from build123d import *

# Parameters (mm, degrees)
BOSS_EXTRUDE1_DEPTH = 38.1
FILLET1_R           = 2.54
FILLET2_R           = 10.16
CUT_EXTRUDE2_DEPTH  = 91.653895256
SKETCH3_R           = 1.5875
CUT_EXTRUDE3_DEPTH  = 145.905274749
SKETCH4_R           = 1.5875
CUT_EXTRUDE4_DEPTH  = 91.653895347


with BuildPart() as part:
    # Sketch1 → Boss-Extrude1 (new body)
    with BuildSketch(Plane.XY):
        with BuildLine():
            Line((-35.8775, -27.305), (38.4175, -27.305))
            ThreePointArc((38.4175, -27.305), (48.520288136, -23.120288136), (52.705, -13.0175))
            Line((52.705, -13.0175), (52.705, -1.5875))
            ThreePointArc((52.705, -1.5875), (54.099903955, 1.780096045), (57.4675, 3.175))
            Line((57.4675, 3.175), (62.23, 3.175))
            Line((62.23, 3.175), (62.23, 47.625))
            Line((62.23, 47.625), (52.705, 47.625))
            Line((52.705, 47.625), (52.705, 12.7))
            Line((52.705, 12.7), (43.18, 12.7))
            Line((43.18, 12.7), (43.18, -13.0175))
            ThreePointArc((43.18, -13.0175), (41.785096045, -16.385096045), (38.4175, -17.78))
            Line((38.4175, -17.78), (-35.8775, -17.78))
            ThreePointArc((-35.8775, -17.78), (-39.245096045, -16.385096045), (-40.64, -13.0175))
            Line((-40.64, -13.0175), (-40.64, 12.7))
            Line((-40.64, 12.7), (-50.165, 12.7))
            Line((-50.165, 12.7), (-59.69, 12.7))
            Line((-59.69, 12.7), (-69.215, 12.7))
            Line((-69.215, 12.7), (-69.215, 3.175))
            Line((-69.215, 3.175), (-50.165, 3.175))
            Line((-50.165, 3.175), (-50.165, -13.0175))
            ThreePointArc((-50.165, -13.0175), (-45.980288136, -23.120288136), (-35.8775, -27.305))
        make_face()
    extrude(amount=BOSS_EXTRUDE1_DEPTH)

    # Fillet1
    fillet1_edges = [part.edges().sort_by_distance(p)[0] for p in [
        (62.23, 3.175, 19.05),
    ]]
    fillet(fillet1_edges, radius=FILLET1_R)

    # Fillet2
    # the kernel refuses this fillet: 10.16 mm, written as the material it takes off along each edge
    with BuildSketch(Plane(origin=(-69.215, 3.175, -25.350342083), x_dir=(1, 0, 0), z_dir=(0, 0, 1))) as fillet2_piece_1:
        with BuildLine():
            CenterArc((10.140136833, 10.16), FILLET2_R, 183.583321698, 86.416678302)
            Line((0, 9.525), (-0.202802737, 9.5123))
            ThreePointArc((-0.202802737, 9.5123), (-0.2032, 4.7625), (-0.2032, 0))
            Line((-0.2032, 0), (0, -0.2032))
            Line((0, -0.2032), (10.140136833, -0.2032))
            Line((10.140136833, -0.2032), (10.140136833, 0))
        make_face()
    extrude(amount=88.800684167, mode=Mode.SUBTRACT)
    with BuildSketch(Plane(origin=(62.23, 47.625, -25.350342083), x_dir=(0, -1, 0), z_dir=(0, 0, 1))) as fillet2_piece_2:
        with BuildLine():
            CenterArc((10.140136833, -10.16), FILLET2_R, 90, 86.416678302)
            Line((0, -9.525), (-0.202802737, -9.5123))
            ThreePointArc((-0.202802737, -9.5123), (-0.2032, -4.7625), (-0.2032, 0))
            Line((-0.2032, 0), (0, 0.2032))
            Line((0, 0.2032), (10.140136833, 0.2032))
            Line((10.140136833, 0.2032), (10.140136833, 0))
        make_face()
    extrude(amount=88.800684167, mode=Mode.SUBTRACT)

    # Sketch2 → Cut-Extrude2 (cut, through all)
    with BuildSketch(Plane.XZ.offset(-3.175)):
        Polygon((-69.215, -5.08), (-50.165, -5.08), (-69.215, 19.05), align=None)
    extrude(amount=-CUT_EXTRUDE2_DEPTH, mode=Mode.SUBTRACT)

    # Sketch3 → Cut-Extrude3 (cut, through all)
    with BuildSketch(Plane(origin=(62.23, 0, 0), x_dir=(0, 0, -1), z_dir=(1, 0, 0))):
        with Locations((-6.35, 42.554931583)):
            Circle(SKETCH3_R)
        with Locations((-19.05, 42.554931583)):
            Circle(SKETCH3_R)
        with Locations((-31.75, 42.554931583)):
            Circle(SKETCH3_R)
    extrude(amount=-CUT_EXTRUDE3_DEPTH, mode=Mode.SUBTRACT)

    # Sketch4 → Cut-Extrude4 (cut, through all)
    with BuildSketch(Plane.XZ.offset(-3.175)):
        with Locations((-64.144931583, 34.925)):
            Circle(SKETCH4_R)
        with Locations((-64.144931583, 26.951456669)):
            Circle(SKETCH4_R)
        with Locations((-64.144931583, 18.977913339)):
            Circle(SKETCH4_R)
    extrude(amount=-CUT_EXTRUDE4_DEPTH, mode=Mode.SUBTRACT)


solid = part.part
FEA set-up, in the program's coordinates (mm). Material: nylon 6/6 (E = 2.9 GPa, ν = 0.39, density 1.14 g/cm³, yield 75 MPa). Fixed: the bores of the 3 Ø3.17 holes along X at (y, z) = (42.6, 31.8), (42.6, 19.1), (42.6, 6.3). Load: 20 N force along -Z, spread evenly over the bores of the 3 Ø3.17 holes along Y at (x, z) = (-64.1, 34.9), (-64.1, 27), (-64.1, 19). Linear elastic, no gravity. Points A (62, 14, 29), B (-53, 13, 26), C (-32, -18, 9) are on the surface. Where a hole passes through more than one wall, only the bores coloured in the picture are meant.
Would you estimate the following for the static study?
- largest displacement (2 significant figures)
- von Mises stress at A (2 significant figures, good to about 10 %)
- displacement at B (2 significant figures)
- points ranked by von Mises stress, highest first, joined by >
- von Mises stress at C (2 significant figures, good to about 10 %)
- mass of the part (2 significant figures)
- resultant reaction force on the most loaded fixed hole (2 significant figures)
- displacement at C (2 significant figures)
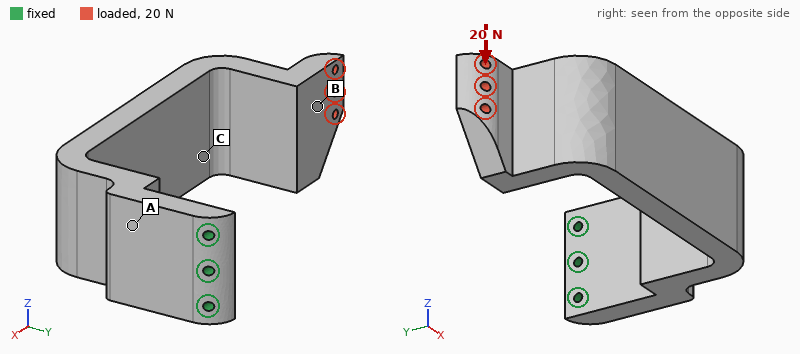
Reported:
1.7 mm
2.9 MPa
1.5 mm
A > C > B
0.98 MPa
87 g
78 N
1.0 mm
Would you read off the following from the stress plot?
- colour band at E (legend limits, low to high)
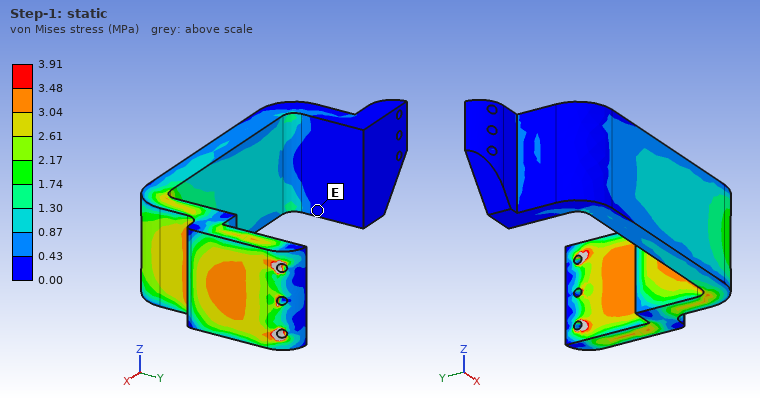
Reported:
0.00 to 0.43 MPa
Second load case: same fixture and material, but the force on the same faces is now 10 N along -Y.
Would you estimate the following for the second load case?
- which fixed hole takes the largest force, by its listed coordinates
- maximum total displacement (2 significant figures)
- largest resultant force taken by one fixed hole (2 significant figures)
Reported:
(42.6, 19.1)
1.7 mm
12 N
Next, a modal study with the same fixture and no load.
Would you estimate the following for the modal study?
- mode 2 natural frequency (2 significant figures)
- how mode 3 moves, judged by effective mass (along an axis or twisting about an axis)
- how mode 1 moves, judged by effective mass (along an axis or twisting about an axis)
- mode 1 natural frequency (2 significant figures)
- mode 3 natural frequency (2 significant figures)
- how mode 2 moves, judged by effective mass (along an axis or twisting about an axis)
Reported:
120 Hz
along X
along Y
82 Hz
250 Hz
along Z
